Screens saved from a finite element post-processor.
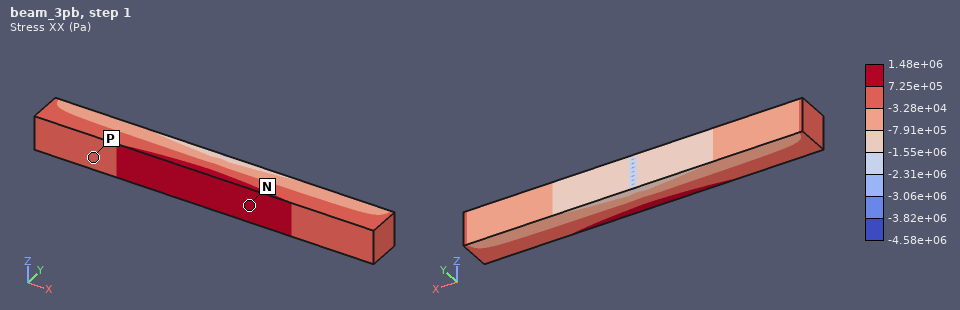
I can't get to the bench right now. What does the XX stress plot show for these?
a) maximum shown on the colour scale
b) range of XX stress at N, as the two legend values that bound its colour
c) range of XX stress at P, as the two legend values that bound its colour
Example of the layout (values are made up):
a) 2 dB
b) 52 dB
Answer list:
a) 1.48e+06 Pa
b) 7.25e+05 to 1.48e+06 Pa
c) -3.28e+04 to 7.25e+05 Pa
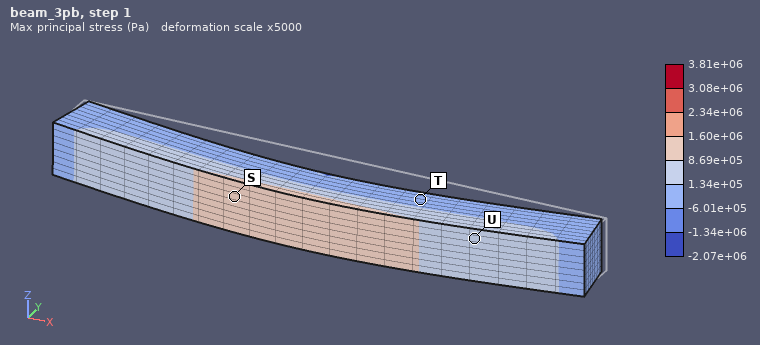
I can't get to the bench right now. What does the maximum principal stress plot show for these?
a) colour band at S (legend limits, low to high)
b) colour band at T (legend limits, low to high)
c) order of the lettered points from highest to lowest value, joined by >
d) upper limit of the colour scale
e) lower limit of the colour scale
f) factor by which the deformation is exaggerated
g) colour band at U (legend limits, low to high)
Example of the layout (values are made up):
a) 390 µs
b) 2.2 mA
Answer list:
a) 8.69e+05 to 1.60e+06 Pa
b) -6.01e+05 to 1.34e+05 Pa
c) S > U > T
d) 3.81e+06 Pa
e) -2.07e+06 Pa
f) 5000
g) 1.34e+05 to 8.69e+05 Pa
